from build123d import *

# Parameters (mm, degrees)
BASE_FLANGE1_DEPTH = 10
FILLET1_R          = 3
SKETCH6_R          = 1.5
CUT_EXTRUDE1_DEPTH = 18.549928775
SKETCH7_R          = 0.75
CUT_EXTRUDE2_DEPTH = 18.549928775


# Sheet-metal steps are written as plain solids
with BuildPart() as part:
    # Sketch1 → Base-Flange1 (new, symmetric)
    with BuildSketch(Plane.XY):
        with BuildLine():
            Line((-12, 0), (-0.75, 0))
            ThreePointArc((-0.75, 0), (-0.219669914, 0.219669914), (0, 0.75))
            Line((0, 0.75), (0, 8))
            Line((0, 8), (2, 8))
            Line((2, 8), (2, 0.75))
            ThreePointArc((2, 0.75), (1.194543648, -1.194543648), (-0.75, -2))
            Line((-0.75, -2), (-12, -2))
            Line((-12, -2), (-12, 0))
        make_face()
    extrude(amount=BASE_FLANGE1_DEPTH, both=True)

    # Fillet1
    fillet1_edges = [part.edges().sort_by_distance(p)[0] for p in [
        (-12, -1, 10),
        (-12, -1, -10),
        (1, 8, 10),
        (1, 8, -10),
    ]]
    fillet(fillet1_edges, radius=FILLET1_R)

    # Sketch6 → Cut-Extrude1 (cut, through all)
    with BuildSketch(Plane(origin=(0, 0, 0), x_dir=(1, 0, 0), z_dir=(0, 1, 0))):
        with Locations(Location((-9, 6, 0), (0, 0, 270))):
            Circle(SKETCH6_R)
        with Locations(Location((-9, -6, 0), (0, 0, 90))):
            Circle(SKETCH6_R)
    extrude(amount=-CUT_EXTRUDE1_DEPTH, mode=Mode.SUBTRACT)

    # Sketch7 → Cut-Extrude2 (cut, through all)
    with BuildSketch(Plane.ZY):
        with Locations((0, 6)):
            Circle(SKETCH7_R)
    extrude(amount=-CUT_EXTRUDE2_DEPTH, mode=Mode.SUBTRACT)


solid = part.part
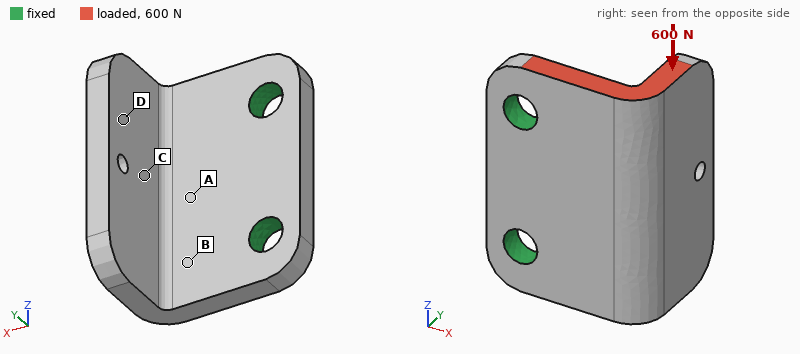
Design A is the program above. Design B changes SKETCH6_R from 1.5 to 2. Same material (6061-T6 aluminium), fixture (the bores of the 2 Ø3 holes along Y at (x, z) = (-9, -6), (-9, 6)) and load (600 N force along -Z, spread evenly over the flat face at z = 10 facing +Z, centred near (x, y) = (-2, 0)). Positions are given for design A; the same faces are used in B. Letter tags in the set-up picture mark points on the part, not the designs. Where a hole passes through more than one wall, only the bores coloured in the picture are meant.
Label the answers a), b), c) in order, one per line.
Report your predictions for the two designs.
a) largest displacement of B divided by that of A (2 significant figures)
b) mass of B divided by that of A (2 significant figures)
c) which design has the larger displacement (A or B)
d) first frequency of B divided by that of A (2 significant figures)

a) 0.87
b) 0.97
c) A
d) 1.1
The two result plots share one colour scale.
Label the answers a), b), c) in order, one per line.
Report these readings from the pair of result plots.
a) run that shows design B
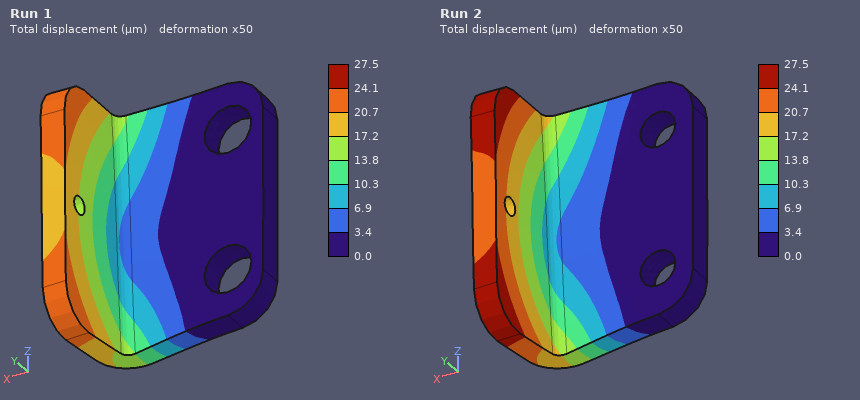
a) Run 1
